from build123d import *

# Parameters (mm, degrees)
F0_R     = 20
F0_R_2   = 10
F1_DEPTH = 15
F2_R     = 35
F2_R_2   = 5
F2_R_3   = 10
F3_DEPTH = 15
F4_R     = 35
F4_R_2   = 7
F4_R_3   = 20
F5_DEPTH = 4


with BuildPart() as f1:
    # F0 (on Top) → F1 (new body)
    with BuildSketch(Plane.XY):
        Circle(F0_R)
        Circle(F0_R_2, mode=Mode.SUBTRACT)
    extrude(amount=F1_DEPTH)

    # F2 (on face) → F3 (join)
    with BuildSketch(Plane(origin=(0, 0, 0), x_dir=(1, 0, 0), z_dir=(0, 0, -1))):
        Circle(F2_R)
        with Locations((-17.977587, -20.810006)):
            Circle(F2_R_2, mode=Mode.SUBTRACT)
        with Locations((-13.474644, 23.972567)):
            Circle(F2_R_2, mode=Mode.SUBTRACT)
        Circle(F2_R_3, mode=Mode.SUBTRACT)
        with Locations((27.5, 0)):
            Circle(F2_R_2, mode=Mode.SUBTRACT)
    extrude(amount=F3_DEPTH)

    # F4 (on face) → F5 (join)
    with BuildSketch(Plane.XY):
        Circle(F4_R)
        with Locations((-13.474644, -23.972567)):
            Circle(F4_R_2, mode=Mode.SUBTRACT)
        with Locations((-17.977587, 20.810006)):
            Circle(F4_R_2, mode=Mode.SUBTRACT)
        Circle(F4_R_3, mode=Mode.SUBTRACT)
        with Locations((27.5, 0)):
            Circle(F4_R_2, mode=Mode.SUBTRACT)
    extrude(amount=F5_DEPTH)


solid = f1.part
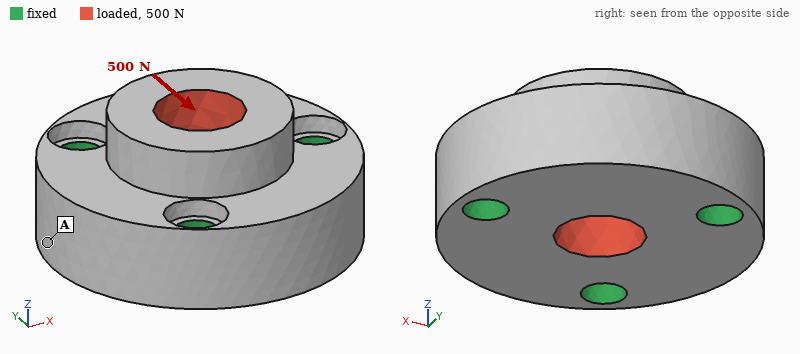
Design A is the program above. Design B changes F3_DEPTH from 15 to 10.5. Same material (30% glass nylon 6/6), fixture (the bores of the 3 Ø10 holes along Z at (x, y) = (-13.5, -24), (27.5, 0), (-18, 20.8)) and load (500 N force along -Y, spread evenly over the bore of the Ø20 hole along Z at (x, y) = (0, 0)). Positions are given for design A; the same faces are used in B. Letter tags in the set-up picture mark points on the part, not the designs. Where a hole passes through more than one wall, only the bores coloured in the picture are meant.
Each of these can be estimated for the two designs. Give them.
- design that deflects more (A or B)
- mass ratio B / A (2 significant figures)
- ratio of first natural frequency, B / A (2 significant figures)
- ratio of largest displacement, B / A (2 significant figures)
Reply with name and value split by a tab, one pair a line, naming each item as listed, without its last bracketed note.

design that deflects more	B
mass ratio B / A	0.79
ratio of first natural frequency, B / A	0.87
ratio of largest displacement, B / A	1.3
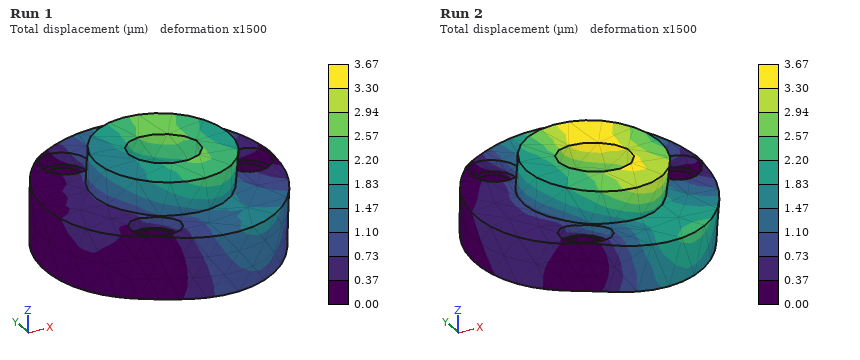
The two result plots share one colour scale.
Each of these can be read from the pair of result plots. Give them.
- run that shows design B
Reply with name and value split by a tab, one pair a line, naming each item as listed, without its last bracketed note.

run that shows design B	Run 2
